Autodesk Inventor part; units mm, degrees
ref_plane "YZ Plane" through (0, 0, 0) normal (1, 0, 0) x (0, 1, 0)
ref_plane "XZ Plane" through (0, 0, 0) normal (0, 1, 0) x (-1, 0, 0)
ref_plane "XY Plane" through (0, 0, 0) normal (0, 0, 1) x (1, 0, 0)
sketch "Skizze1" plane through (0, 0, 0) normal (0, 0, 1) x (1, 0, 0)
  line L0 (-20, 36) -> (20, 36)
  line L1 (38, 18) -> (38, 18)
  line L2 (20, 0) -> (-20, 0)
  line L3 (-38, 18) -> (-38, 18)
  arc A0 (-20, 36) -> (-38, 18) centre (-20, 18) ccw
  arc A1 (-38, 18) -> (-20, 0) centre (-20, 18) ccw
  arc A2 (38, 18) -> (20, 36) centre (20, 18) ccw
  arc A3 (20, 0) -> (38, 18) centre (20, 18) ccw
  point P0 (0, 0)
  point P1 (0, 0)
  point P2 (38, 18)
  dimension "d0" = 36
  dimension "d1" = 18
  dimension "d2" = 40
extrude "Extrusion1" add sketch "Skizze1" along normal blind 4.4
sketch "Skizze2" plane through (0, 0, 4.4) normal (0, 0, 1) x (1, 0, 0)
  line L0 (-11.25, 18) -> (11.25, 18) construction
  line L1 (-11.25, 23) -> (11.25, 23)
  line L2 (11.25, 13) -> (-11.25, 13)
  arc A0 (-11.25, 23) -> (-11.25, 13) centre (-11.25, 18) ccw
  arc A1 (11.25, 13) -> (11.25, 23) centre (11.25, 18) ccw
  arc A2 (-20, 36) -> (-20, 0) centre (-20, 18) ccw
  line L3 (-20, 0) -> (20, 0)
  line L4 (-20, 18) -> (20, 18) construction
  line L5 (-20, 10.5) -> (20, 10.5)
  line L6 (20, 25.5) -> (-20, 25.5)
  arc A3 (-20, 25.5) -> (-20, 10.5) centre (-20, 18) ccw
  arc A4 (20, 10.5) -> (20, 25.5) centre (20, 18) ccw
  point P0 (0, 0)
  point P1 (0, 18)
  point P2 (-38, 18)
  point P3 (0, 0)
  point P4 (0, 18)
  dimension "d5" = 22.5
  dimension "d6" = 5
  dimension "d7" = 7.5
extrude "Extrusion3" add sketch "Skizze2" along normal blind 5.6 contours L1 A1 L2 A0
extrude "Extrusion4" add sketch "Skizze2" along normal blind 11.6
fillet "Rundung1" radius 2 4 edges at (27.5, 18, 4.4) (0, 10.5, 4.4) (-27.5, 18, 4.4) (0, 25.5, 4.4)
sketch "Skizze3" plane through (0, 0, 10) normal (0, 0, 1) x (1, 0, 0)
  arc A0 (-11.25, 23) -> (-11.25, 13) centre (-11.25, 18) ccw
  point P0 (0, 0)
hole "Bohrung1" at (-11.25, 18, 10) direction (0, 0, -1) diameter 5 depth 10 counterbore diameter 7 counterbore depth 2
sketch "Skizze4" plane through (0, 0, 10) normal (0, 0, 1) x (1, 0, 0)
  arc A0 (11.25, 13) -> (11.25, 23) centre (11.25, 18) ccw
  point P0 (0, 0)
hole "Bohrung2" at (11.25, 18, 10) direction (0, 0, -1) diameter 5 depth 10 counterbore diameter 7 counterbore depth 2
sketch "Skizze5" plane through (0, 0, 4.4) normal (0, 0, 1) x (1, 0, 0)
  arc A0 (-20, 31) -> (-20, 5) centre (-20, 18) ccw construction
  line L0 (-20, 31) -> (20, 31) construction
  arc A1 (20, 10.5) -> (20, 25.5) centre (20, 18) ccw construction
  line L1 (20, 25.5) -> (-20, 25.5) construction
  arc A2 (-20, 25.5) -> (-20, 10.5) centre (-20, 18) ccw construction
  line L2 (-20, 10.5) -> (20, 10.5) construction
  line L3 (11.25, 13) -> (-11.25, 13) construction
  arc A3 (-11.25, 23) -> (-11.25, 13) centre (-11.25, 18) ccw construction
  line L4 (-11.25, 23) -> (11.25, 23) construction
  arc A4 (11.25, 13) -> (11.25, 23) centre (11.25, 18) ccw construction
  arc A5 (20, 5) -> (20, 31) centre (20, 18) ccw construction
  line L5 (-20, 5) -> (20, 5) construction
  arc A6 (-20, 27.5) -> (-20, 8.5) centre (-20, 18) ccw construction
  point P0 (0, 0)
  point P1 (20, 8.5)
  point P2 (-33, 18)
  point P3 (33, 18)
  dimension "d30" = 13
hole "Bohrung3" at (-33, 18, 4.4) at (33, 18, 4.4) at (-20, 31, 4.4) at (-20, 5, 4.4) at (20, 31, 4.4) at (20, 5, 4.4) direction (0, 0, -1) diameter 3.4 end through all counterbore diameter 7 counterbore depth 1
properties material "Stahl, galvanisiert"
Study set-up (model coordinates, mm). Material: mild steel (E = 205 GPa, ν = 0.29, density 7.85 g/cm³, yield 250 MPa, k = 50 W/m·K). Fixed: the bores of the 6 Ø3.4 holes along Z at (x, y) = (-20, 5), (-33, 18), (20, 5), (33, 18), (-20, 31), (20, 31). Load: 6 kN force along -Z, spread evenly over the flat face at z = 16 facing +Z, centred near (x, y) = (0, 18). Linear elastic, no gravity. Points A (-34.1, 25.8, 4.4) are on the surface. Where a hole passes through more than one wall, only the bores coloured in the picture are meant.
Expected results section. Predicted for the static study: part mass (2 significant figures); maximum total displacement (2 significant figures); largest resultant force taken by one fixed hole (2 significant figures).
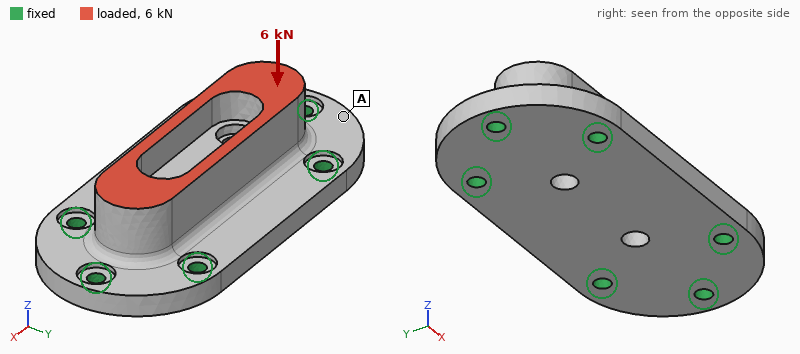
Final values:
140 g
6.9 µm
1.3 kN
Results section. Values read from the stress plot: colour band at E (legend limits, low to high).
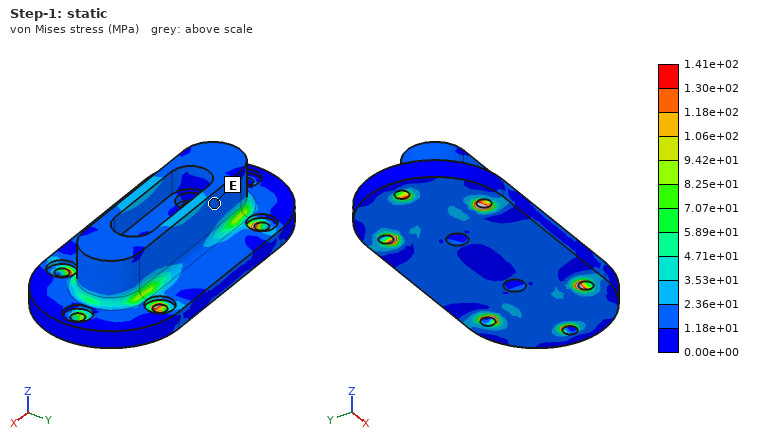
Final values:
1.18e+01 to 2.36e+01 MPa
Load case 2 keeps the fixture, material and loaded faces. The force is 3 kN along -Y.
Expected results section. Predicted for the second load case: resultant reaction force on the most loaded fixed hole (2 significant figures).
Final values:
1.1 kN
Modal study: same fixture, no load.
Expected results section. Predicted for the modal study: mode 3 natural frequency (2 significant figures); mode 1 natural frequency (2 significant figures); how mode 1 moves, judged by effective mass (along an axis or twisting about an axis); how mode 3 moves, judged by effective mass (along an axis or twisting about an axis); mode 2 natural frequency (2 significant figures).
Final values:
25 kHz
14 kHz
along Z
along Y
18 kHz
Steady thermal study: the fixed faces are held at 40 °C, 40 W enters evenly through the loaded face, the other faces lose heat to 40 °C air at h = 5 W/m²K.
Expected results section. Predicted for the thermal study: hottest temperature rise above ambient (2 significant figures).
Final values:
36 K
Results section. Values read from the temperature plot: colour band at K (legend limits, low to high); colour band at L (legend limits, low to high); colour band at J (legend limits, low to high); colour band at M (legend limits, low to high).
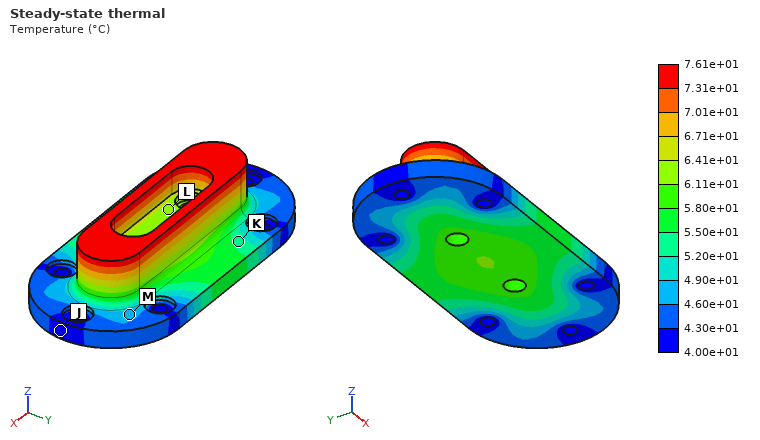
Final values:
5.20e+01 to 5.50e+01 °C
6.11e+01 to 6.41e+01 °C
4.00e+01 to 4.30e+01 °C
4.60e+01 to 4.90e+01 °C
